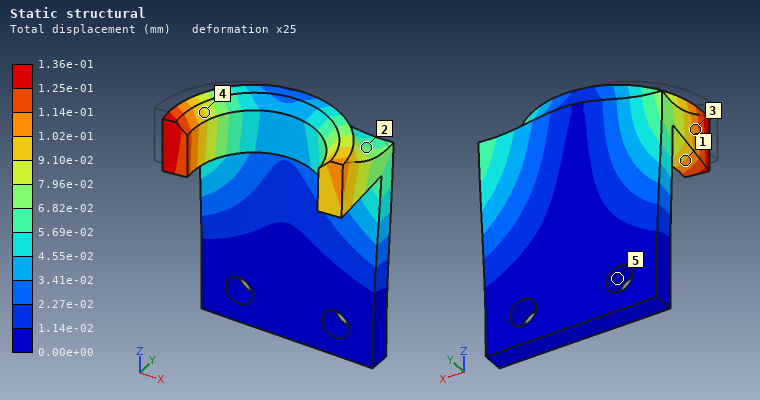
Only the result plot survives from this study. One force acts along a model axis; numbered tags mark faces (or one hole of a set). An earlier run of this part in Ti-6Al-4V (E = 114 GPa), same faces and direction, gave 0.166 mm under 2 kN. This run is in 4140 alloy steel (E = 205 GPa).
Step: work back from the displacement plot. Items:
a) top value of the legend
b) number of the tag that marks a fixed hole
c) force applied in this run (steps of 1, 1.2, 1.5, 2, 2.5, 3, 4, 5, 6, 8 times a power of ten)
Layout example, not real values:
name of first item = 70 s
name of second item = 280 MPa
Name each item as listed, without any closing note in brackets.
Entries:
top value of the legend = 1.36e-01 mm
number of the tag that marks a fixed hole = 5
force applied in this run = 3 kN
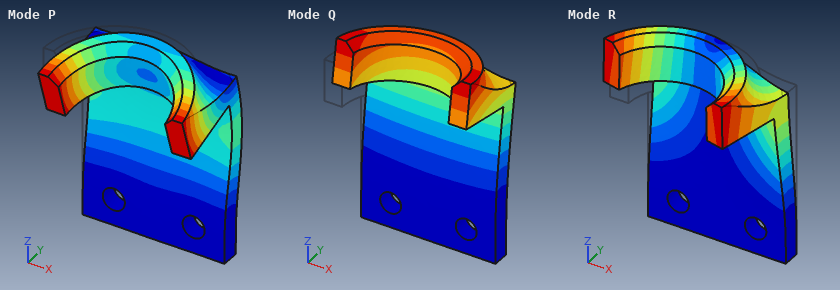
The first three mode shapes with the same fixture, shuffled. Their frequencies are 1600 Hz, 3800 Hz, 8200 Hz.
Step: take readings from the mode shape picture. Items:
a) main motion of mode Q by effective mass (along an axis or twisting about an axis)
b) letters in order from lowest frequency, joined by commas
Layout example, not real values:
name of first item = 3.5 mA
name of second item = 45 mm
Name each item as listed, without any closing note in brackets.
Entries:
main motion of mode Q by effective mass = along Y
letters in order from lowest frequency, joined by commas = Q, R, P
